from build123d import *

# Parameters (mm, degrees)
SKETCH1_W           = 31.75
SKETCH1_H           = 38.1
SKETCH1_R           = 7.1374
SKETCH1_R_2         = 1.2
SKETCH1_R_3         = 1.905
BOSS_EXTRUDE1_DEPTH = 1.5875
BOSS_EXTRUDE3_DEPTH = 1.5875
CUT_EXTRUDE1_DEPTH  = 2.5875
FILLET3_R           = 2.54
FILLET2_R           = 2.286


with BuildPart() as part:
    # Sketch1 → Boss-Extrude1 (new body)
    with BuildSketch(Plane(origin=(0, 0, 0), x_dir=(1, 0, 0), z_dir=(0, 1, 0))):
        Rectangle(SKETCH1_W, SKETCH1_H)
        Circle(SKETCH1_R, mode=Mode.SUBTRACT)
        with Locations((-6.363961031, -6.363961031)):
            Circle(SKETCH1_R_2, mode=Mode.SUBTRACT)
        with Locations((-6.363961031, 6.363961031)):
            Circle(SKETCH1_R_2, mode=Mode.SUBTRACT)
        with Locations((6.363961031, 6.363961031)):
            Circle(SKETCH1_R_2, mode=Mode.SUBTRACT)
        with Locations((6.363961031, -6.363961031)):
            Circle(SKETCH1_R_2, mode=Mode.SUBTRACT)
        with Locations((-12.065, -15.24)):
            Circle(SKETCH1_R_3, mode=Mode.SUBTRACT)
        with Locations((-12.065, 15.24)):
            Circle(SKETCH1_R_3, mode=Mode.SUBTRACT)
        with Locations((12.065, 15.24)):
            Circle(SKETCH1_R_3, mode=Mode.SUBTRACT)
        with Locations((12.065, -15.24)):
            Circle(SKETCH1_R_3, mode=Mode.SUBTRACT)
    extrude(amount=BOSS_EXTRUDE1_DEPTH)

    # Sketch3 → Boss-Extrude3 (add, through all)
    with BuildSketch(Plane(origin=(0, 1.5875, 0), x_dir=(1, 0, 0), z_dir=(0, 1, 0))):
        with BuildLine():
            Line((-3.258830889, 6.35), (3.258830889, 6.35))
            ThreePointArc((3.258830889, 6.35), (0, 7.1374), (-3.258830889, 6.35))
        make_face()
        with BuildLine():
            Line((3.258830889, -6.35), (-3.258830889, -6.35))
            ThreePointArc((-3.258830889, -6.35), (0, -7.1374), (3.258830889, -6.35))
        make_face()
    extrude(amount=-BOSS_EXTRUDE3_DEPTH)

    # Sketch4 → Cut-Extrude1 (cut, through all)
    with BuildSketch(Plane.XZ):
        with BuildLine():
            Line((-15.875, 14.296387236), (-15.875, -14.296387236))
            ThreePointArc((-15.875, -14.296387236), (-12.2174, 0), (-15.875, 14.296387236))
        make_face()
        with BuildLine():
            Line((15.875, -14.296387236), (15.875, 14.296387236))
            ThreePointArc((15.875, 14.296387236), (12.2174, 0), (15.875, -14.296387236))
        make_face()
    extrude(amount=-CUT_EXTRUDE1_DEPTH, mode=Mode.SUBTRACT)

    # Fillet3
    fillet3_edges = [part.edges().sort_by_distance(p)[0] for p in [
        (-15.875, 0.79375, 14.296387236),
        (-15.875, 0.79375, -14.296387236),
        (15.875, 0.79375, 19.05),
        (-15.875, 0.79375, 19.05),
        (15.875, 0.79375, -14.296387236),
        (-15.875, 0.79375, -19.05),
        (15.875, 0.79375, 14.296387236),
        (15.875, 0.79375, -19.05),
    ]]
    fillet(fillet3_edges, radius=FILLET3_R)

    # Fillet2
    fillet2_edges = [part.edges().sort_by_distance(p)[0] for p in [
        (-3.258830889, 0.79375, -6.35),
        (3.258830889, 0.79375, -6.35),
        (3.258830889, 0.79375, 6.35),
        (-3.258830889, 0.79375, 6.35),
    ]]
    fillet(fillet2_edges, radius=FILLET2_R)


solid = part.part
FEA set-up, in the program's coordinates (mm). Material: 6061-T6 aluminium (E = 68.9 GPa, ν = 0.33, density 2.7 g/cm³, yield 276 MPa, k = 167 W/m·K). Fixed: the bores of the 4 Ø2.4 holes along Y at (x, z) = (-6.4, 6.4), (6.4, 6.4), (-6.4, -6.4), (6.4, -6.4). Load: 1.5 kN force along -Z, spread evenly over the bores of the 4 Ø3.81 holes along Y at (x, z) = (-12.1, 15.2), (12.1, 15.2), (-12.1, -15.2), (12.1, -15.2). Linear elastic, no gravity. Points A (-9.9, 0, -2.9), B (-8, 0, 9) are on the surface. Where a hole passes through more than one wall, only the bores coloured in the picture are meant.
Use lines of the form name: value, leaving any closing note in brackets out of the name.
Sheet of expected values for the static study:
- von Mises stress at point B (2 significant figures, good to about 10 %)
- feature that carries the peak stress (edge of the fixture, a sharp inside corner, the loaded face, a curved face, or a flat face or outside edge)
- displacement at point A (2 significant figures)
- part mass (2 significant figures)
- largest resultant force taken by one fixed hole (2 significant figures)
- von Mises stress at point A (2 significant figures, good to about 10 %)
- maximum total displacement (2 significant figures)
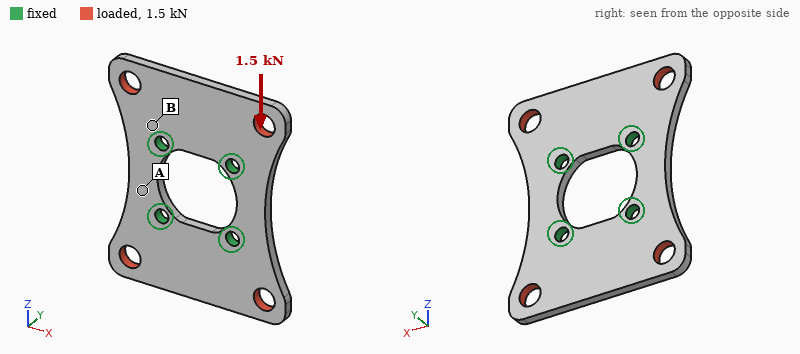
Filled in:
von Mises stress at point B: 36 MPa
feature that carries the peak stress: edge of the fixture
displacement at point A: 2.1 µm
part mass: 3.6 g
largest resultant force taken by one fixed hole: 380 N
von Mises stress at point A: 17 MPa
maximum total displacement: 12 µm
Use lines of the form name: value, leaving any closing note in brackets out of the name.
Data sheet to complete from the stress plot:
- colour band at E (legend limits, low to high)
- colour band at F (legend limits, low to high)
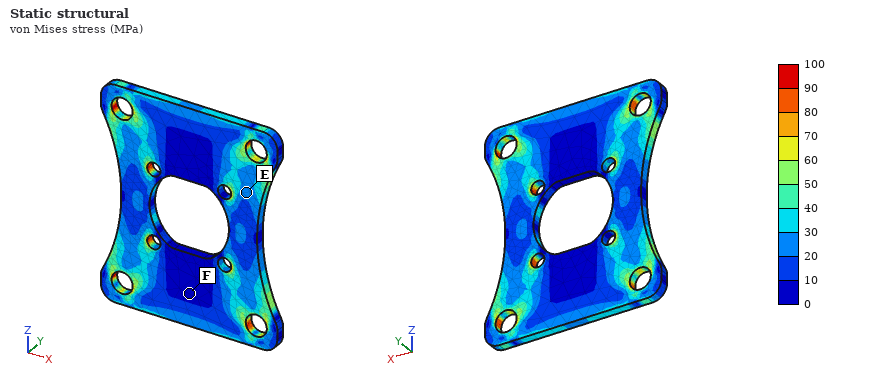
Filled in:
colour band at E: 20 to 30 MPa
colour band at F: 0 to 10 MPa
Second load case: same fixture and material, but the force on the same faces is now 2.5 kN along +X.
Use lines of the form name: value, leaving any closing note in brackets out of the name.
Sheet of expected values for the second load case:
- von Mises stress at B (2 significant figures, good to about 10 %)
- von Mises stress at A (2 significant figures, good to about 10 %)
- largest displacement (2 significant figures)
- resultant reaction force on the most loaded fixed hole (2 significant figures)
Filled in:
von Mises stress at B: 63 MPa
von Mises stress at A: 32 MPa
largest displacement: 30 µm
resultant reaction force on the most loaded fixed hole: 680 N
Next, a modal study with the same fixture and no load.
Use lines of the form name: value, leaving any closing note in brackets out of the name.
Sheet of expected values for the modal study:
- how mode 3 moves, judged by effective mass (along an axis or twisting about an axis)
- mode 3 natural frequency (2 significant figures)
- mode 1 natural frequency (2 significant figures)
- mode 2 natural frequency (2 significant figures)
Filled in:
how mode 3 moves, judged by effective mass: twisting about Z
mode 3 natural frequency: 9600 Hz
mode 1 natural frequency: 7500 Hz
mode 2 natural frequency: 7600 Hz
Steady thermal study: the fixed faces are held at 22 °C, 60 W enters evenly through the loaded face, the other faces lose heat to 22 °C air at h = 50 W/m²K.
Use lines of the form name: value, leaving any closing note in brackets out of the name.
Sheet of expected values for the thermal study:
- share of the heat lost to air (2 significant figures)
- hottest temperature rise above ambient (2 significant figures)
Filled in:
share of the heat lost to air: 4.4 %
hottest temperature rise above ambient: 70 K
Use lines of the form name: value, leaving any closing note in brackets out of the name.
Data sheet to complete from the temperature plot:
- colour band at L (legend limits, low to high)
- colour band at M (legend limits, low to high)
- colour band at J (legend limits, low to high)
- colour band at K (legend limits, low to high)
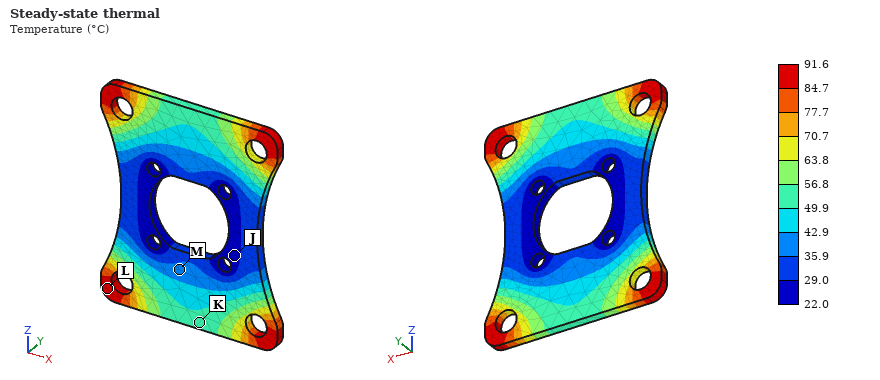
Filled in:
colour band at L: 84.7 to 91.6 °C
colour band at M: 35.9 to 42.9 °C
colour band at J: 22.0 to 29.0 °C
colour band at K: 49.9 to 56.8 °C
